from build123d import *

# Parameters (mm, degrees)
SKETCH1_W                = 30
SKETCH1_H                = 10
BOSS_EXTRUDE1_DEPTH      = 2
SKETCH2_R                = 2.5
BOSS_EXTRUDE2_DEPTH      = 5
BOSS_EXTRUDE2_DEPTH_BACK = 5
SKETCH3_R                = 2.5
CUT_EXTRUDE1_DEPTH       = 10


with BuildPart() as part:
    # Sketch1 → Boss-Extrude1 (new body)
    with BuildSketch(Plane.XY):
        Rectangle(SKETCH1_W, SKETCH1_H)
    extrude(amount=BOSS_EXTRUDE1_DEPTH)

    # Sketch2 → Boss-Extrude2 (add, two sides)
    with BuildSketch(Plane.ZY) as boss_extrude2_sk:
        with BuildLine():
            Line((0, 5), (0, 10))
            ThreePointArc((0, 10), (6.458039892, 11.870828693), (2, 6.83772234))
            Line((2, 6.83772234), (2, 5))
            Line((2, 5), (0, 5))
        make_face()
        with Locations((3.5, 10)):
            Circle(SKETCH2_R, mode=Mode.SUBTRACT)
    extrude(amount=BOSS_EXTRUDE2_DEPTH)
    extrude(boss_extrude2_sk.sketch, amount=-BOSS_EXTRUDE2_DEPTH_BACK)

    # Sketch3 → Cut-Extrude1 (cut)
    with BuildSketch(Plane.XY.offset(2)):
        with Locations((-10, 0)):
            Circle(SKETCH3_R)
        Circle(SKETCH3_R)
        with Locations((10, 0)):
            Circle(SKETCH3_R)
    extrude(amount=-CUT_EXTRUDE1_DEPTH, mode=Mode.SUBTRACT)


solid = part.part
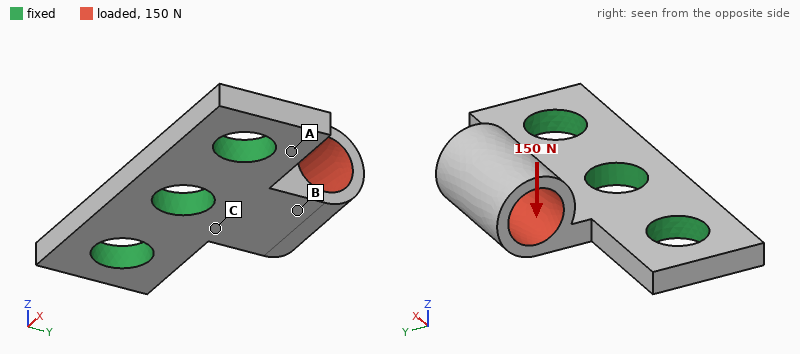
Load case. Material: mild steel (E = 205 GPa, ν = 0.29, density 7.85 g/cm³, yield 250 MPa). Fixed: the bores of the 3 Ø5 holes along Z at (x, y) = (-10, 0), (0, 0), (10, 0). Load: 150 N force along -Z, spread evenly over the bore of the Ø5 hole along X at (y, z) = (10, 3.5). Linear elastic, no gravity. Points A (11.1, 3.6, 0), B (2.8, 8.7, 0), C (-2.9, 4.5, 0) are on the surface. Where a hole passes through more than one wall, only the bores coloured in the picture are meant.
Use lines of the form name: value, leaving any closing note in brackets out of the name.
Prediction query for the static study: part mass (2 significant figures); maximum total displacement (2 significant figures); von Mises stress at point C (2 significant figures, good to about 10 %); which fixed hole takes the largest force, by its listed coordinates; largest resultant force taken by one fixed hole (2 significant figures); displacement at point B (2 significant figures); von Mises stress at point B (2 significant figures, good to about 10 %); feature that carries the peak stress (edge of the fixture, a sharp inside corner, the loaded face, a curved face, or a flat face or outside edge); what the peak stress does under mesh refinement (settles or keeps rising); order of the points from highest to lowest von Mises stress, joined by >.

part mass: 5.7 g
maximum total displacement: 33 µm
von Mises stress at point C: 100 MPa
which fixed hole takes the largest force, by its listed coordinates: (0, 0)
largest resultant force taken by one fixed hole: 140 N
displacement at point B: 13 µm
von Mises stress at point B: 57 MPa
feature that carries the peak stress: edge of the fixture
what the peak stress does under mesh refinement: keeps rising
order of the points from highest to lowest von Mises stress, joined by >: C > B > A
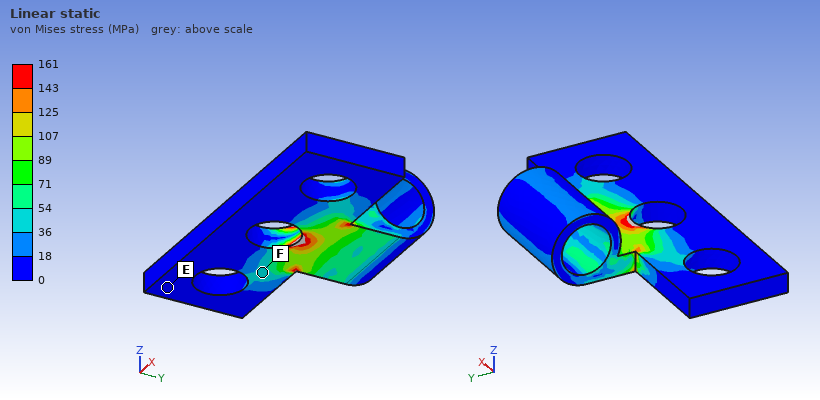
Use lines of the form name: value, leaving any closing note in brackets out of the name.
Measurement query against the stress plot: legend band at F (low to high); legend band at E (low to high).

legend band at F: 36 to 54 MPa
legend band at E: 0 to 18 MPa
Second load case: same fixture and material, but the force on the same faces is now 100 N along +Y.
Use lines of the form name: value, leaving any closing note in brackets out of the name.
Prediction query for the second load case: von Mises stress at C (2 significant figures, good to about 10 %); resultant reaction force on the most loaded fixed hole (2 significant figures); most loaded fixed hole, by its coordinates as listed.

von Mises stress at C: 27 MPa
resultant reaction force on the most loaded fixed hole: 78 N
most loaded fixed hole, by its coordinates as listed: (0, 0)
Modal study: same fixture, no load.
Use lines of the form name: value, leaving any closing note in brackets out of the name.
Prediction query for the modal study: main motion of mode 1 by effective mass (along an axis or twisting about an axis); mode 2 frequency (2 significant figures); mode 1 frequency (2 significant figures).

main motion of mode 1 by effective mass: along Z
mode 2 frequency: 22 kHz
mode 1 frequency: 9200 Hz
